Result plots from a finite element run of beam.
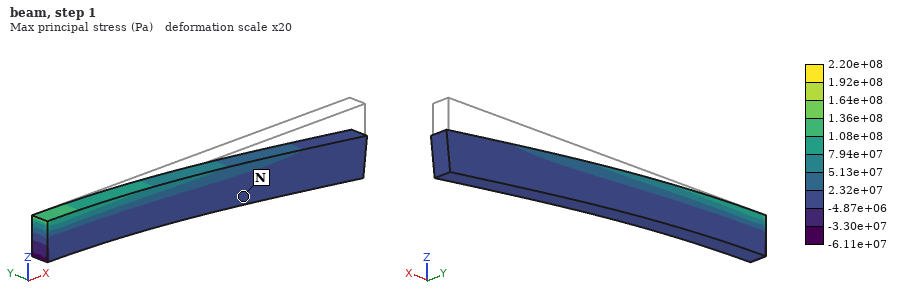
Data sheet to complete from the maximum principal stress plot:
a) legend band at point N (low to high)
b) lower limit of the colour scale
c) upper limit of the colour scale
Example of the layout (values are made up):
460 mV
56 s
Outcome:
-4.87e+06 to 2.32e+07 Pa
-6.11e+07 Pa
2.20e+08 Pa
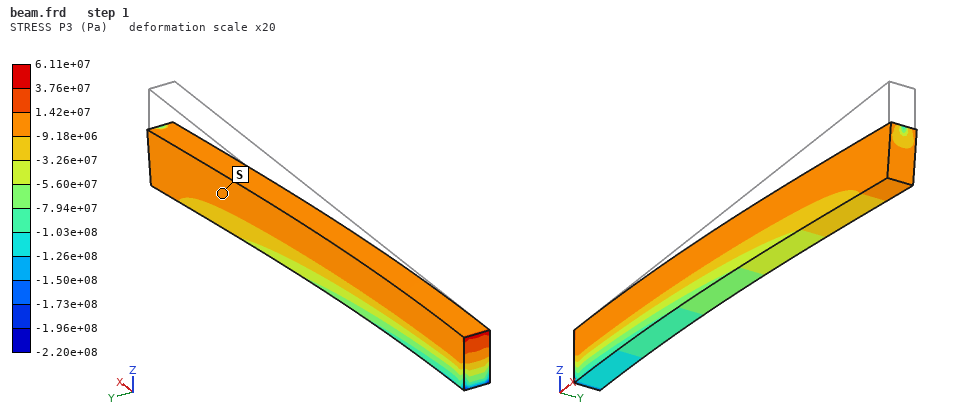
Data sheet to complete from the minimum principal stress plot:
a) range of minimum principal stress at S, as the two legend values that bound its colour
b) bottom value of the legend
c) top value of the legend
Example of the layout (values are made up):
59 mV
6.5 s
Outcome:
-9.18e+06 to 1.42e+07 Pa
-2.20e+08 Pa
6.11e+07 Pa
